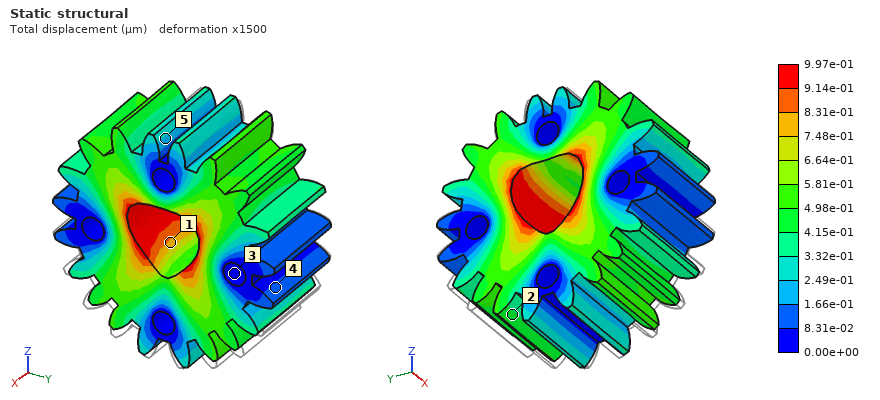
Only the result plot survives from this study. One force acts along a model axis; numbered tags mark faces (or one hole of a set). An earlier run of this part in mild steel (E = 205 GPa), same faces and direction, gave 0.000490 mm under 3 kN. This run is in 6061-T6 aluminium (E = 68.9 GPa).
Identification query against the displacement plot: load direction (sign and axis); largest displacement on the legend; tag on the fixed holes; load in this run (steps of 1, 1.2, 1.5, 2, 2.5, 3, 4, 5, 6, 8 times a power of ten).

+Z
9.97e-01 µm
3
2 kN
